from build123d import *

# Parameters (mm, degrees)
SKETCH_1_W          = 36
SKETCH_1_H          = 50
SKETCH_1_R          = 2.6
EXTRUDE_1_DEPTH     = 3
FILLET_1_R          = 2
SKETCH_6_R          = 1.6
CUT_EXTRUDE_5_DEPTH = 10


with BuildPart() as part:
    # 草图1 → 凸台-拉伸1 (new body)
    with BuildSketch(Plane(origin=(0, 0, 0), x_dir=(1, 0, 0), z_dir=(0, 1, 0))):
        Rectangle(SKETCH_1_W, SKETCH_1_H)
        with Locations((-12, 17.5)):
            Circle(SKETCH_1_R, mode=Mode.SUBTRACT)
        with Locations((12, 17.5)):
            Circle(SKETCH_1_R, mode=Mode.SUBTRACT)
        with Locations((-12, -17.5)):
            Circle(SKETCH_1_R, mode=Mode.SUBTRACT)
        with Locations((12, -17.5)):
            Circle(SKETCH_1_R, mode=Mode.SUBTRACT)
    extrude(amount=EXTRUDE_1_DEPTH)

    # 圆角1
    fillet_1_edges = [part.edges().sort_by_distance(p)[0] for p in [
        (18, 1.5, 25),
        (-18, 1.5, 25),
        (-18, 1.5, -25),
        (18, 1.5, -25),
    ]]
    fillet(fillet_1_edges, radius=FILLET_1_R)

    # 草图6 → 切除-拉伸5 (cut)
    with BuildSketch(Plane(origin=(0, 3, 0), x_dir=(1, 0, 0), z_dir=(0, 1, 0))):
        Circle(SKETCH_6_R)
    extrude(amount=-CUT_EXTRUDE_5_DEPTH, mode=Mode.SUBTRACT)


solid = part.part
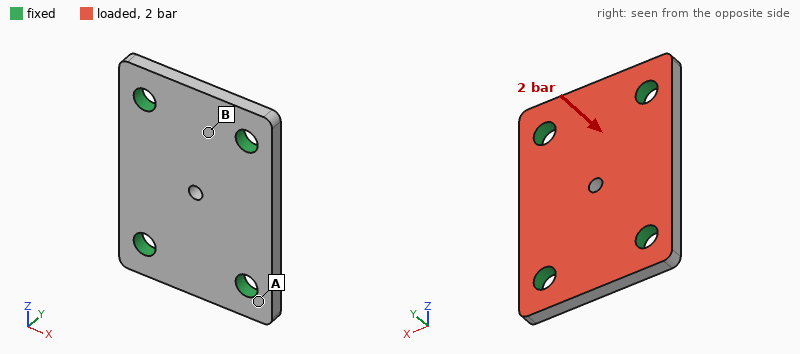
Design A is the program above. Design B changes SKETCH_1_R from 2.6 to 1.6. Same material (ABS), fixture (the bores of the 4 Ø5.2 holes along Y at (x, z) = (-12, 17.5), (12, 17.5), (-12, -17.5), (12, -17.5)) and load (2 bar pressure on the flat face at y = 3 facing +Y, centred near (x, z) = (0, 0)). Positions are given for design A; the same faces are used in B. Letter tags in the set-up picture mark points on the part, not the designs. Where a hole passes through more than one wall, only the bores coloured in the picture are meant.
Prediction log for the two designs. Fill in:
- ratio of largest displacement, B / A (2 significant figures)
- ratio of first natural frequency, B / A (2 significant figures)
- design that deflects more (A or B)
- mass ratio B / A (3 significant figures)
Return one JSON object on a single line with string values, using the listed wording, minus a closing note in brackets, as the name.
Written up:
{"ratio of largest displacement, B / A": "1.3", "ratio of first natural frequency, B / A": "0.86", "design that deflects more": "B", "mass ratio B / A": "1.03"}
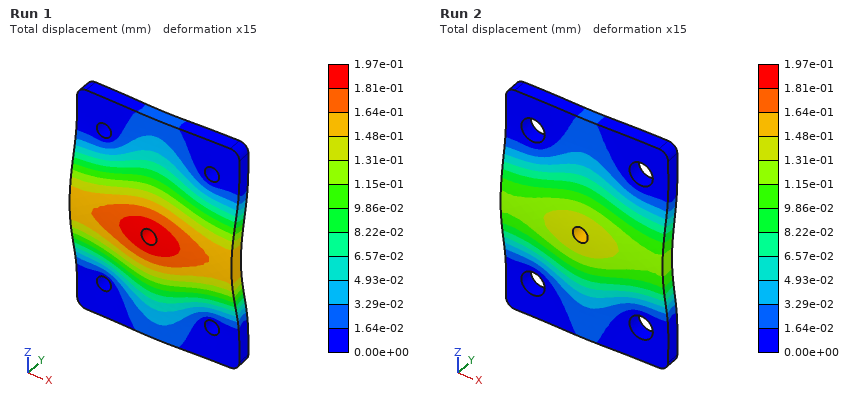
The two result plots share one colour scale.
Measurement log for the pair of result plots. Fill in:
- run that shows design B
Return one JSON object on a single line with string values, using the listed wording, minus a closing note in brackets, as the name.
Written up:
{"run that shows design B": "Run 1"}
